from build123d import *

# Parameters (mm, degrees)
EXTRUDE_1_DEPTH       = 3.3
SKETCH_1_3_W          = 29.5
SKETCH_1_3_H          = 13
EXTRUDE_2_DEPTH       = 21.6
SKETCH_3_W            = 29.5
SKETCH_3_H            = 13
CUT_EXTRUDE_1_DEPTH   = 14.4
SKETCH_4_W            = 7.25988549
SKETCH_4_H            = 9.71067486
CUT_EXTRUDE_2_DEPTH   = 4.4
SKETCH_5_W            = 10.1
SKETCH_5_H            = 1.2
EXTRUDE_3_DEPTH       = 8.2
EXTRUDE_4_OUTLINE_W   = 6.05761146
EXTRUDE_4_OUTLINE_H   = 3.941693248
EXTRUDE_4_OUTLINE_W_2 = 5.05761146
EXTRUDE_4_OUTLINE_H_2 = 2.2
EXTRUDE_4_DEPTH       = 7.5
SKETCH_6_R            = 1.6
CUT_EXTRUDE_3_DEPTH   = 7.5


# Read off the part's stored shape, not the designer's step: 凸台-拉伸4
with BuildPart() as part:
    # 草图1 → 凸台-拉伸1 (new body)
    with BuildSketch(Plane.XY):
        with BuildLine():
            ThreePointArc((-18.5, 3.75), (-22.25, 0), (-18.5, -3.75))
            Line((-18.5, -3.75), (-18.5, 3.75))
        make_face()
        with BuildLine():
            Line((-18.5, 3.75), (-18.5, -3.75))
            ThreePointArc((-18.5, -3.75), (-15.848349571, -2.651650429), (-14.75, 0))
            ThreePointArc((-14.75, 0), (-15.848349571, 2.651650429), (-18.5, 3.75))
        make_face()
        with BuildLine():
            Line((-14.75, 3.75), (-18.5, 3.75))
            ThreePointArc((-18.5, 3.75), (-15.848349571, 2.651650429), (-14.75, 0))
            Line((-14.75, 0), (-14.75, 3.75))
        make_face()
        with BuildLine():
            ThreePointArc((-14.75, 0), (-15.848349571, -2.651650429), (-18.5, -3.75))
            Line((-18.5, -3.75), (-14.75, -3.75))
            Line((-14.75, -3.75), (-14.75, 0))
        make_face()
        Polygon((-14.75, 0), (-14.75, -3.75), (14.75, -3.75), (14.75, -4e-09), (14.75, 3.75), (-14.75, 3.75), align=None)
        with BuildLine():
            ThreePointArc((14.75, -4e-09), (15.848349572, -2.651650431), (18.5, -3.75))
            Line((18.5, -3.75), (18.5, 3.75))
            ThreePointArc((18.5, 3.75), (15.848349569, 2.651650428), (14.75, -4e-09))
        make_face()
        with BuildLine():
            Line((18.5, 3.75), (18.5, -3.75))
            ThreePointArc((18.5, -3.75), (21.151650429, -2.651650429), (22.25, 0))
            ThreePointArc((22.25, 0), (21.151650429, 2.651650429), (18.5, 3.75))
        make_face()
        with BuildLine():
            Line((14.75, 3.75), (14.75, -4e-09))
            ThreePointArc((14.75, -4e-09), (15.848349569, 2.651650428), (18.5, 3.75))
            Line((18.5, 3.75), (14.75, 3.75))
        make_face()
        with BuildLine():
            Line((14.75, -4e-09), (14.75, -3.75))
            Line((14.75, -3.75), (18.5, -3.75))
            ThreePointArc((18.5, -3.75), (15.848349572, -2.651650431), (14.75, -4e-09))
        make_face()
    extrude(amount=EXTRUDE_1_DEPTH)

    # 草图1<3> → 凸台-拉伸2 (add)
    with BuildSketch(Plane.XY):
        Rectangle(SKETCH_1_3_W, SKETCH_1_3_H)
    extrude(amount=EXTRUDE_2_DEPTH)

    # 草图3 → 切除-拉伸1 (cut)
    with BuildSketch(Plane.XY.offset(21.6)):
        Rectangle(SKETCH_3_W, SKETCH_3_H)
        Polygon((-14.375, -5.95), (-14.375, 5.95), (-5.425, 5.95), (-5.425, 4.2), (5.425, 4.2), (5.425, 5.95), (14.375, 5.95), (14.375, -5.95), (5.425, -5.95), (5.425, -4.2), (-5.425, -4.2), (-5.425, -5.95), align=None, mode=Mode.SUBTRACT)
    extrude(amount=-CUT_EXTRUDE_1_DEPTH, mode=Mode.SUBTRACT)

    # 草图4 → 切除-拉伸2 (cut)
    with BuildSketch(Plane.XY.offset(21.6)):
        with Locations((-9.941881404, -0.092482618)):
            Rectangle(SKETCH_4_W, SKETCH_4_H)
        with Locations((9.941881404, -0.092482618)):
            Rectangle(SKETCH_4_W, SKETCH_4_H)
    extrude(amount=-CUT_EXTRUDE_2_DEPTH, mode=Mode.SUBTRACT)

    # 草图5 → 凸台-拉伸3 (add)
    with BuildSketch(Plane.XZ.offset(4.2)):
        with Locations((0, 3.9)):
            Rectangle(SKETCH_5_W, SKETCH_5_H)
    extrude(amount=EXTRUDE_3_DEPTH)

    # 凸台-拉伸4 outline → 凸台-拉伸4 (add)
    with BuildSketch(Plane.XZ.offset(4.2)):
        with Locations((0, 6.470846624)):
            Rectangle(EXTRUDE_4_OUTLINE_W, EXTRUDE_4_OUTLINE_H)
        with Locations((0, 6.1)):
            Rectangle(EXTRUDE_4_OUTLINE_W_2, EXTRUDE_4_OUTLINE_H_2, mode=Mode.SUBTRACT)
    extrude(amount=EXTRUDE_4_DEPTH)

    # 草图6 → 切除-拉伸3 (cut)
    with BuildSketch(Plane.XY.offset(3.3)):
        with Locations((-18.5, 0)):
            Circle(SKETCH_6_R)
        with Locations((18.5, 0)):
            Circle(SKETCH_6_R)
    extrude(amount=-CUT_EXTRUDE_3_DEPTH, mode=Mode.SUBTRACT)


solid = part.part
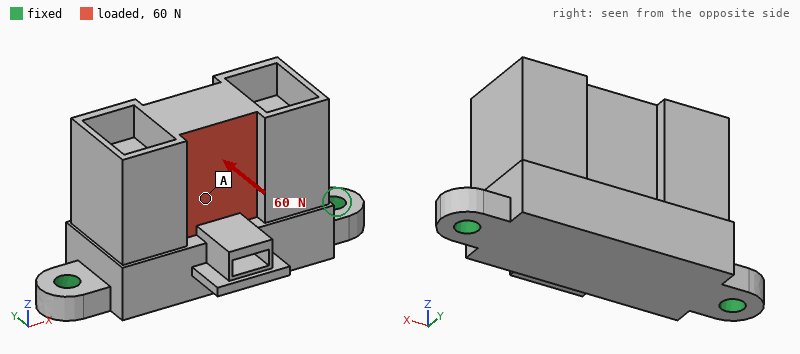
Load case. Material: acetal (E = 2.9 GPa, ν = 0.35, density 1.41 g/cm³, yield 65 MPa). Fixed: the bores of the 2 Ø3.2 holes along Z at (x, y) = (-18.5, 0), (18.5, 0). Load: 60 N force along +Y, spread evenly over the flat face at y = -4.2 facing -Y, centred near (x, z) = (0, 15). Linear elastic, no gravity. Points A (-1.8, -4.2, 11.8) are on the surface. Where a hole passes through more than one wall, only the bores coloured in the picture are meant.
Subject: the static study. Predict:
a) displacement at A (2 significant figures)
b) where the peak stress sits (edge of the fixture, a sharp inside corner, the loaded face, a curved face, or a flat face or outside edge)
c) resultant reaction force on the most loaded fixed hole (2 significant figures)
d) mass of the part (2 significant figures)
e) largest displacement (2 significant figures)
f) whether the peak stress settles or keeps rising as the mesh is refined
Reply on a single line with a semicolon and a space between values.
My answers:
0.20 mm; edge of the fixture; 30 N; 9.8 g; 0.37 mm; keeps rising
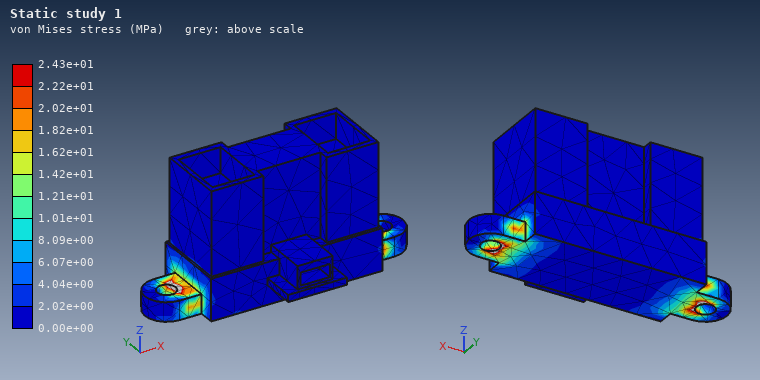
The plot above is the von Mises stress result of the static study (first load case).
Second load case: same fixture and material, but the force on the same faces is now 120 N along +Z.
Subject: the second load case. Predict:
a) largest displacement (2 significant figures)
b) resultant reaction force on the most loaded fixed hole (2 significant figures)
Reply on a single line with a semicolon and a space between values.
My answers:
0.24 mm; 69 N
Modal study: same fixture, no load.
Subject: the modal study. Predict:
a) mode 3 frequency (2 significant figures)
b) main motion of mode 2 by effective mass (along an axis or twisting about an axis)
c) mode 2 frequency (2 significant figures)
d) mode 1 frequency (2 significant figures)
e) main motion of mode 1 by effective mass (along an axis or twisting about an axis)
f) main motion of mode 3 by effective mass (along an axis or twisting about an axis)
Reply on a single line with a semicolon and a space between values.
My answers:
4900 Hz; along Z; 4000 Hz; 1100 Hz; along Y; along X
